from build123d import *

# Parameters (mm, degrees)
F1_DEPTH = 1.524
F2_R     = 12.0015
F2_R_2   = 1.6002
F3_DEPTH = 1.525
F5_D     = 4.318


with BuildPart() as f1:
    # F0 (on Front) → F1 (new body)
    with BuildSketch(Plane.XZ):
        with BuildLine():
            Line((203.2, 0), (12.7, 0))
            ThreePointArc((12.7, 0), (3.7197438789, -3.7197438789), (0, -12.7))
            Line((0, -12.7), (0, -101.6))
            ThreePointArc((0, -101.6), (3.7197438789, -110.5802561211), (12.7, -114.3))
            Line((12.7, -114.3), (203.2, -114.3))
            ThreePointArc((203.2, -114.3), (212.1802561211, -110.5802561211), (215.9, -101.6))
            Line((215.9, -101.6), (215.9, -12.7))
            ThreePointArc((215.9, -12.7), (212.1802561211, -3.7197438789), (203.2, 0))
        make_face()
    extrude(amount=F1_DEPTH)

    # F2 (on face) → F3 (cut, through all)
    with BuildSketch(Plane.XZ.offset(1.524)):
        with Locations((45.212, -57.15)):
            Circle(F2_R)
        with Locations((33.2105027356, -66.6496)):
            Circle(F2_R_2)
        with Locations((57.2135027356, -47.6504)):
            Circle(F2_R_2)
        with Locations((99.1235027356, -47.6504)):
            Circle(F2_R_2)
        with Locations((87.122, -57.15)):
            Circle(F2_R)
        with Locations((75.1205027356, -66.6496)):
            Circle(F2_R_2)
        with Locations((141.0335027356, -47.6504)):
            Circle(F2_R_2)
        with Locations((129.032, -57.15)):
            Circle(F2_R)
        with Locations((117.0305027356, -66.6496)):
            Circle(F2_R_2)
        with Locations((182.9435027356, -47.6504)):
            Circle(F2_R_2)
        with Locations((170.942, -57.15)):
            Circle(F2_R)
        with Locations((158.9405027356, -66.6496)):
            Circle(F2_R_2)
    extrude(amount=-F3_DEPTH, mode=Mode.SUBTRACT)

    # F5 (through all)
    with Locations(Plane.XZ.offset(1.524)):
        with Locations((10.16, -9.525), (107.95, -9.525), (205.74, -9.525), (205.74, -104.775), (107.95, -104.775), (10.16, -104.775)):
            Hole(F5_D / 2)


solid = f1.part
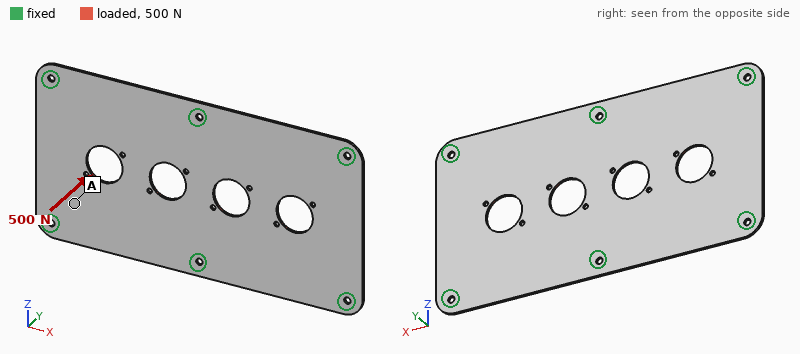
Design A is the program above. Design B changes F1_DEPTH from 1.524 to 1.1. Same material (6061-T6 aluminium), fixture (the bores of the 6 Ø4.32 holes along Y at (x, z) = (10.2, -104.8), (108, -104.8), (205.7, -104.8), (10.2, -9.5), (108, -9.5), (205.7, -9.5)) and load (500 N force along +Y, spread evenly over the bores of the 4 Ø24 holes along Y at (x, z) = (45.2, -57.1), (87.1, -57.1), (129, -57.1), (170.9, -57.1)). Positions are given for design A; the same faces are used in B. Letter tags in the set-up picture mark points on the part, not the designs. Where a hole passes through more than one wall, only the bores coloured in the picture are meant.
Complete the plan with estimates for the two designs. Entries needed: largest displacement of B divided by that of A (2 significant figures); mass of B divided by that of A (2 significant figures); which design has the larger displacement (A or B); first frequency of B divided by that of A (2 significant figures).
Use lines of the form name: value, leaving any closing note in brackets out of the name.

largest displacement of B divided by that of A: 2.6
mass of B divided by that of A: 0.72
which design has the larger displacement: B
first frequency of B divided by that of A: 0.73
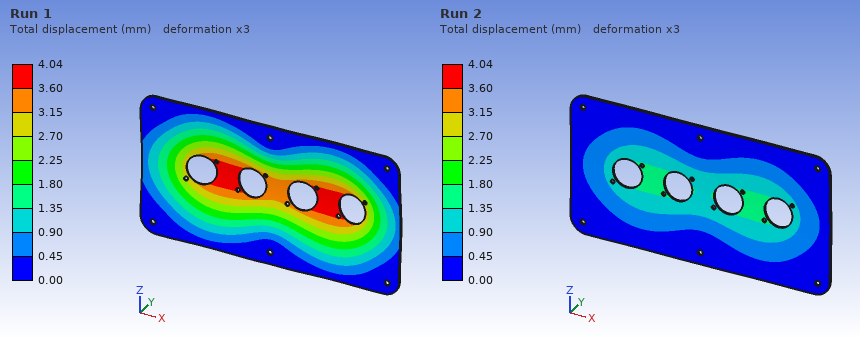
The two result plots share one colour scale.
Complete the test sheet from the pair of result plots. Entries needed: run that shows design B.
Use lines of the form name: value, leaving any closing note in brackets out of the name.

run that shows design B: Run 1
